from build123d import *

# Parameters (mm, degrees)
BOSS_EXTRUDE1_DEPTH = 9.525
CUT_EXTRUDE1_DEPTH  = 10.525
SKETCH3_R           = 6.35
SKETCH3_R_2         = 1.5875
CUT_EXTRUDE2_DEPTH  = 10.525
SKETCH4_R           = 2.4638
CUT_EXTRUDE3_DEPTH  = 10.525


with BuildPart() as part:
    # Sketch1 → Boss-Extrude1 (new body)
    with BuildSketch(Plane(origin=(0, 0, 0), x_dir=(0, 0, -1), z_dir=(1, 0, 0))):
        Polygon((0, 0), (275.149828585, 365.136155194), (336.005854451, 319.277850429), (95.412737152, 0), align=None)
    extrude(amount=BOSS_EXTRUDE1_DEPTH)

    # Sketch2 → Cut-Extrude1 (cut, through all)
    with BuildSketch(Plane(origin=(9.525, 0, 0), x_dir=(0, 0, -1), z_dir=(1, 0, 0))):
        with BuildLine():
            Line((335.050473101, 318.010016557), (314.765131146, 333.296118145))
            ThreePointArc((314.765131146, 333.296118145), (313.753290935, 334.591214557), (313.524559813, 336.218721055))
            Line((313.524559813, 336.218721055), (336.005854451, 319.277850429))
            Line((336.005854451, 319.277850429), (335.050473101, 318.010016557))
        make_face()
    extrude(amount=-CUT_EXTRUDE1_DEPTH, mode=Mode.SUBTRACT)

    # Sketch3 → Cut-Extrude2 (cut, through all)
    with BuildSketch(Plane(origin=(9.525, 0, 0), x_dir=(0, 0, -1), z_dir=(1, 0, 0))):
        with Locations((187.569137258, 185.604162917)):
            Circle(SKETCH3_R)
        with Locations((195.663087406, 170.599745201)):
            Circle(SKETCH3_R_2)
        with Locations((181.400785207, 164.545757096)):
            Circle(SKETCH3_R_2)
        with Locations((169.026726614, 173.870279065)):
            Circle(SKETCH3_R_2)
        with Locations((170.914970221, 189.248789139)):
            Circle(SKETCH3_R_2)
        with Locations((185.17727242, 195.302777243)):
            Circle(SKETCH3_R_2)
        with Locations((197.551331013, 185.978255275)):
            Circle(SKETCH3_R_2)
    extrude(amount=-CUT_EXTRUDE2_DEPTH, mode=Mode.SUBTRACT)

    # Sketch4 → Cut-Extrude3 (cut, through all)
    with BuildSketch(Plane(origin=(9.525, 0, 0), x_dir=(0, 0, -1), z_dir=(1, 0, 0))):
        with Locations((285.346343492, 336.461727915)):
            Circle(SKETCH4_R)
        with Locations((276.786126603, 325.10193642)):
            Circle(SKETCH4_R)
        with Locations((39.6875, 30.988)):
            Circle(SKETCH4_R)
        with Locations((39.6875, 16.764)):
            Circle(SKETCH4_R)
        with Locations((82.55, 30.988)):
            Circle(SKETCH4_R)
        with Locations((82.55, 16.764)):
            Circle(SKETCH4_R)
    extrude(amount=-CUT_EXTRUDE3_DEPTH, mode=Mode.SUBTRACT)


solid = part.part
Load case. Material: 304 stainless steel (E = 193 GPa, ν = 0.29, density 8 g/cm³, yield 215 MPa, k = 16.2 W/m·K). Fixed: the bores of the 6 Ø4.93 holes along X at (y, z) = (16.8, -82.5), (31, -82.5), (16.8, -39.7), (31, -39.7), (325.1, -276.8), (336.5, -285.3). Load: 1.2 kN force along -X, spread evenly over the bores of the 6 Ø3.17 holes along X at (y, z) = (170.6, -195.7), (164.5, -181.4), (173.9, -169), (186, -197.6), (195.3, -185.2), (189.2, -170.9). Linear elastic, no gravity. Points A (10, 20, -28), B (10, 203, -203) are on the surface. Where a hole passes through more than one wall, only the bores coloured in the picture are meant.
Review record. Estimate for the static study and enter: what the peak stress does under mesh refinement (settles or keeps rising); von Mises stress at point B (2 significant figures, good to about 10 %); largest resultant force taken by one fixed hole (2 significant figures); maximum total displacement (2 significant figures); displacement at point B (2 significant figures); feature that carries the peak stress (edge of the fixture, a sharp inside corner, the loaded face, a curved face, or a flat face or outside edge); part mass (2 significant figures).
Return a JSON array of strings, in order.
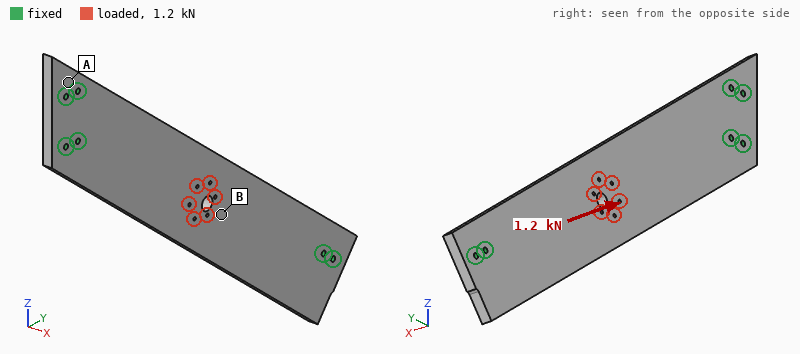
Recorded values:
["keeps rising", "26 MPa", "2.1 kN", "0.29 mm", "0.27 mm", "edge of the fixture", "2.5 kg"]
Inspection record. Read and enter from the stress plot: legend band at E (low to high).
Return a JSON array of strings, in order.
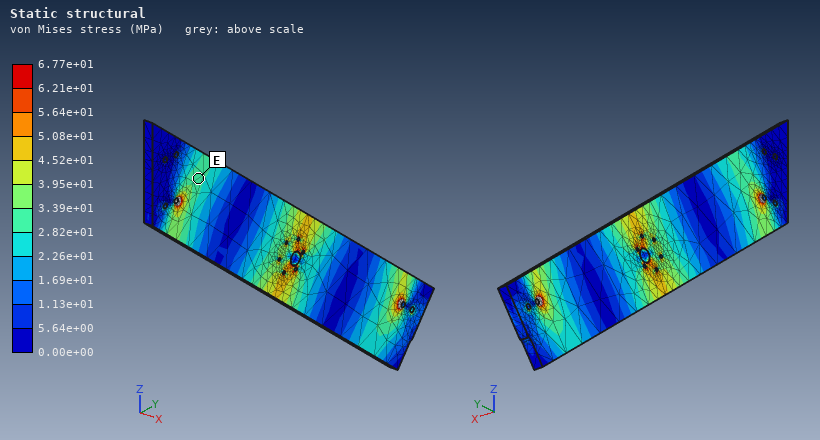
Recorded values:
["2.82e+01 to 3.39e+01 MPa"]
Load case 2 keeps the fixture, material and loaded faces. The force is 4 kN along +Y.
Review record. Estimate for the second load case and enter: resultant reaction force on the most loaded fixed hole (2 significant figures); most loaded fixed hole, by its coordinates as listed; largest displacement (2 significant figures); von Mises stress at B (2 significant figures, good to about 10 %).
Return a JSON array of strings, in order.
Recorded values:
["3.0 kN", "(325.1, -276.8)", "19 µm", "5.4 MPa"]
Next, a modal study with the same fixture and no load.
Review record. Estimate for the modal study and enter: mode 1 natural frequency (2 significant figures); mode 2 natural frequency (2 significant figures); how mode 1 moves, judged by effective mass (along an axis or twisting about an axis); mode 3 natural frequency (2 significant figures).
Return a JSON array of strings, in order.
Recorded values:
["360 Hz", "930 Hz", "along X", "1100 Hz"]
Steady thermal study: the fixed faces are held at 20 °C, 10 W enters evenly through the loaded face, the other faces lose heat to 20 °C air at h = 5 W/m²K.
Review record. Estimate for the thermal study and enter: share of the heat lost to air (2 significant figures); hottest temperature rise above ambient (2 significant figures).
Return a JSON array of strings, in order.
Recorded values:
["62 %", "46 K"]
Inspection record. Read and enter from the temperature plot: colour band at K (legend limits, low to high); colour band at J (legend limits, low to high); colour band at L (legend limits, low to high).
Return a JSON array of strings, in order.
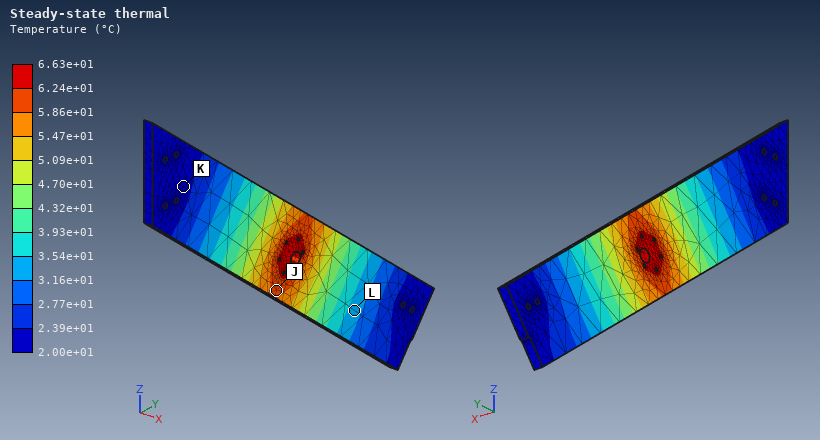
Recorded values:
["2.00e+01 to 2.39e+01 °C", "5.86e+01 to 6.24e+01 °C", "3.16e+01 to 3.54e+01 °C"]
